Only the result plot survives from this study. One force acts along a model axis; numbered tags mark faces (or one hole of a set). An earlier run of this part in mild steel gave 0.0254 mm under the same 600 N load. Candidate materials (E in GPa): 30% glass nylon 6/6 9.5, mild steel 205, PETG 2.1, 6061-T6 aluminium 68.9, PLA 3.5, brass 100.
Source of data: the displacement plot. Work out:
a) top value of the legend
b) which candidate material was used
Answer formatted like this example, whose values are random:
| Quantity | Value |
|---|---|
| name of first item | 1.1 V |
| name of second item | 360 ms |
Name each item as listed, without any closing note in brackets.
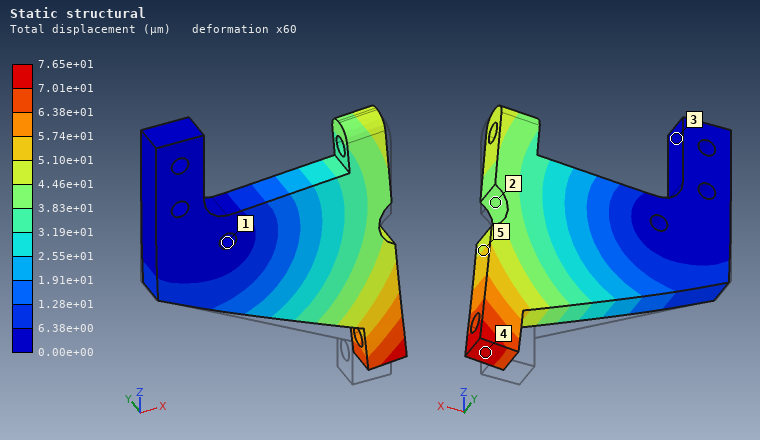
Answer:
| Quantity | Value |
|---|---|
| top value of the legend | 7.65e+01 µm |
| which candidate material was used | 6061-T6 aluminium |
